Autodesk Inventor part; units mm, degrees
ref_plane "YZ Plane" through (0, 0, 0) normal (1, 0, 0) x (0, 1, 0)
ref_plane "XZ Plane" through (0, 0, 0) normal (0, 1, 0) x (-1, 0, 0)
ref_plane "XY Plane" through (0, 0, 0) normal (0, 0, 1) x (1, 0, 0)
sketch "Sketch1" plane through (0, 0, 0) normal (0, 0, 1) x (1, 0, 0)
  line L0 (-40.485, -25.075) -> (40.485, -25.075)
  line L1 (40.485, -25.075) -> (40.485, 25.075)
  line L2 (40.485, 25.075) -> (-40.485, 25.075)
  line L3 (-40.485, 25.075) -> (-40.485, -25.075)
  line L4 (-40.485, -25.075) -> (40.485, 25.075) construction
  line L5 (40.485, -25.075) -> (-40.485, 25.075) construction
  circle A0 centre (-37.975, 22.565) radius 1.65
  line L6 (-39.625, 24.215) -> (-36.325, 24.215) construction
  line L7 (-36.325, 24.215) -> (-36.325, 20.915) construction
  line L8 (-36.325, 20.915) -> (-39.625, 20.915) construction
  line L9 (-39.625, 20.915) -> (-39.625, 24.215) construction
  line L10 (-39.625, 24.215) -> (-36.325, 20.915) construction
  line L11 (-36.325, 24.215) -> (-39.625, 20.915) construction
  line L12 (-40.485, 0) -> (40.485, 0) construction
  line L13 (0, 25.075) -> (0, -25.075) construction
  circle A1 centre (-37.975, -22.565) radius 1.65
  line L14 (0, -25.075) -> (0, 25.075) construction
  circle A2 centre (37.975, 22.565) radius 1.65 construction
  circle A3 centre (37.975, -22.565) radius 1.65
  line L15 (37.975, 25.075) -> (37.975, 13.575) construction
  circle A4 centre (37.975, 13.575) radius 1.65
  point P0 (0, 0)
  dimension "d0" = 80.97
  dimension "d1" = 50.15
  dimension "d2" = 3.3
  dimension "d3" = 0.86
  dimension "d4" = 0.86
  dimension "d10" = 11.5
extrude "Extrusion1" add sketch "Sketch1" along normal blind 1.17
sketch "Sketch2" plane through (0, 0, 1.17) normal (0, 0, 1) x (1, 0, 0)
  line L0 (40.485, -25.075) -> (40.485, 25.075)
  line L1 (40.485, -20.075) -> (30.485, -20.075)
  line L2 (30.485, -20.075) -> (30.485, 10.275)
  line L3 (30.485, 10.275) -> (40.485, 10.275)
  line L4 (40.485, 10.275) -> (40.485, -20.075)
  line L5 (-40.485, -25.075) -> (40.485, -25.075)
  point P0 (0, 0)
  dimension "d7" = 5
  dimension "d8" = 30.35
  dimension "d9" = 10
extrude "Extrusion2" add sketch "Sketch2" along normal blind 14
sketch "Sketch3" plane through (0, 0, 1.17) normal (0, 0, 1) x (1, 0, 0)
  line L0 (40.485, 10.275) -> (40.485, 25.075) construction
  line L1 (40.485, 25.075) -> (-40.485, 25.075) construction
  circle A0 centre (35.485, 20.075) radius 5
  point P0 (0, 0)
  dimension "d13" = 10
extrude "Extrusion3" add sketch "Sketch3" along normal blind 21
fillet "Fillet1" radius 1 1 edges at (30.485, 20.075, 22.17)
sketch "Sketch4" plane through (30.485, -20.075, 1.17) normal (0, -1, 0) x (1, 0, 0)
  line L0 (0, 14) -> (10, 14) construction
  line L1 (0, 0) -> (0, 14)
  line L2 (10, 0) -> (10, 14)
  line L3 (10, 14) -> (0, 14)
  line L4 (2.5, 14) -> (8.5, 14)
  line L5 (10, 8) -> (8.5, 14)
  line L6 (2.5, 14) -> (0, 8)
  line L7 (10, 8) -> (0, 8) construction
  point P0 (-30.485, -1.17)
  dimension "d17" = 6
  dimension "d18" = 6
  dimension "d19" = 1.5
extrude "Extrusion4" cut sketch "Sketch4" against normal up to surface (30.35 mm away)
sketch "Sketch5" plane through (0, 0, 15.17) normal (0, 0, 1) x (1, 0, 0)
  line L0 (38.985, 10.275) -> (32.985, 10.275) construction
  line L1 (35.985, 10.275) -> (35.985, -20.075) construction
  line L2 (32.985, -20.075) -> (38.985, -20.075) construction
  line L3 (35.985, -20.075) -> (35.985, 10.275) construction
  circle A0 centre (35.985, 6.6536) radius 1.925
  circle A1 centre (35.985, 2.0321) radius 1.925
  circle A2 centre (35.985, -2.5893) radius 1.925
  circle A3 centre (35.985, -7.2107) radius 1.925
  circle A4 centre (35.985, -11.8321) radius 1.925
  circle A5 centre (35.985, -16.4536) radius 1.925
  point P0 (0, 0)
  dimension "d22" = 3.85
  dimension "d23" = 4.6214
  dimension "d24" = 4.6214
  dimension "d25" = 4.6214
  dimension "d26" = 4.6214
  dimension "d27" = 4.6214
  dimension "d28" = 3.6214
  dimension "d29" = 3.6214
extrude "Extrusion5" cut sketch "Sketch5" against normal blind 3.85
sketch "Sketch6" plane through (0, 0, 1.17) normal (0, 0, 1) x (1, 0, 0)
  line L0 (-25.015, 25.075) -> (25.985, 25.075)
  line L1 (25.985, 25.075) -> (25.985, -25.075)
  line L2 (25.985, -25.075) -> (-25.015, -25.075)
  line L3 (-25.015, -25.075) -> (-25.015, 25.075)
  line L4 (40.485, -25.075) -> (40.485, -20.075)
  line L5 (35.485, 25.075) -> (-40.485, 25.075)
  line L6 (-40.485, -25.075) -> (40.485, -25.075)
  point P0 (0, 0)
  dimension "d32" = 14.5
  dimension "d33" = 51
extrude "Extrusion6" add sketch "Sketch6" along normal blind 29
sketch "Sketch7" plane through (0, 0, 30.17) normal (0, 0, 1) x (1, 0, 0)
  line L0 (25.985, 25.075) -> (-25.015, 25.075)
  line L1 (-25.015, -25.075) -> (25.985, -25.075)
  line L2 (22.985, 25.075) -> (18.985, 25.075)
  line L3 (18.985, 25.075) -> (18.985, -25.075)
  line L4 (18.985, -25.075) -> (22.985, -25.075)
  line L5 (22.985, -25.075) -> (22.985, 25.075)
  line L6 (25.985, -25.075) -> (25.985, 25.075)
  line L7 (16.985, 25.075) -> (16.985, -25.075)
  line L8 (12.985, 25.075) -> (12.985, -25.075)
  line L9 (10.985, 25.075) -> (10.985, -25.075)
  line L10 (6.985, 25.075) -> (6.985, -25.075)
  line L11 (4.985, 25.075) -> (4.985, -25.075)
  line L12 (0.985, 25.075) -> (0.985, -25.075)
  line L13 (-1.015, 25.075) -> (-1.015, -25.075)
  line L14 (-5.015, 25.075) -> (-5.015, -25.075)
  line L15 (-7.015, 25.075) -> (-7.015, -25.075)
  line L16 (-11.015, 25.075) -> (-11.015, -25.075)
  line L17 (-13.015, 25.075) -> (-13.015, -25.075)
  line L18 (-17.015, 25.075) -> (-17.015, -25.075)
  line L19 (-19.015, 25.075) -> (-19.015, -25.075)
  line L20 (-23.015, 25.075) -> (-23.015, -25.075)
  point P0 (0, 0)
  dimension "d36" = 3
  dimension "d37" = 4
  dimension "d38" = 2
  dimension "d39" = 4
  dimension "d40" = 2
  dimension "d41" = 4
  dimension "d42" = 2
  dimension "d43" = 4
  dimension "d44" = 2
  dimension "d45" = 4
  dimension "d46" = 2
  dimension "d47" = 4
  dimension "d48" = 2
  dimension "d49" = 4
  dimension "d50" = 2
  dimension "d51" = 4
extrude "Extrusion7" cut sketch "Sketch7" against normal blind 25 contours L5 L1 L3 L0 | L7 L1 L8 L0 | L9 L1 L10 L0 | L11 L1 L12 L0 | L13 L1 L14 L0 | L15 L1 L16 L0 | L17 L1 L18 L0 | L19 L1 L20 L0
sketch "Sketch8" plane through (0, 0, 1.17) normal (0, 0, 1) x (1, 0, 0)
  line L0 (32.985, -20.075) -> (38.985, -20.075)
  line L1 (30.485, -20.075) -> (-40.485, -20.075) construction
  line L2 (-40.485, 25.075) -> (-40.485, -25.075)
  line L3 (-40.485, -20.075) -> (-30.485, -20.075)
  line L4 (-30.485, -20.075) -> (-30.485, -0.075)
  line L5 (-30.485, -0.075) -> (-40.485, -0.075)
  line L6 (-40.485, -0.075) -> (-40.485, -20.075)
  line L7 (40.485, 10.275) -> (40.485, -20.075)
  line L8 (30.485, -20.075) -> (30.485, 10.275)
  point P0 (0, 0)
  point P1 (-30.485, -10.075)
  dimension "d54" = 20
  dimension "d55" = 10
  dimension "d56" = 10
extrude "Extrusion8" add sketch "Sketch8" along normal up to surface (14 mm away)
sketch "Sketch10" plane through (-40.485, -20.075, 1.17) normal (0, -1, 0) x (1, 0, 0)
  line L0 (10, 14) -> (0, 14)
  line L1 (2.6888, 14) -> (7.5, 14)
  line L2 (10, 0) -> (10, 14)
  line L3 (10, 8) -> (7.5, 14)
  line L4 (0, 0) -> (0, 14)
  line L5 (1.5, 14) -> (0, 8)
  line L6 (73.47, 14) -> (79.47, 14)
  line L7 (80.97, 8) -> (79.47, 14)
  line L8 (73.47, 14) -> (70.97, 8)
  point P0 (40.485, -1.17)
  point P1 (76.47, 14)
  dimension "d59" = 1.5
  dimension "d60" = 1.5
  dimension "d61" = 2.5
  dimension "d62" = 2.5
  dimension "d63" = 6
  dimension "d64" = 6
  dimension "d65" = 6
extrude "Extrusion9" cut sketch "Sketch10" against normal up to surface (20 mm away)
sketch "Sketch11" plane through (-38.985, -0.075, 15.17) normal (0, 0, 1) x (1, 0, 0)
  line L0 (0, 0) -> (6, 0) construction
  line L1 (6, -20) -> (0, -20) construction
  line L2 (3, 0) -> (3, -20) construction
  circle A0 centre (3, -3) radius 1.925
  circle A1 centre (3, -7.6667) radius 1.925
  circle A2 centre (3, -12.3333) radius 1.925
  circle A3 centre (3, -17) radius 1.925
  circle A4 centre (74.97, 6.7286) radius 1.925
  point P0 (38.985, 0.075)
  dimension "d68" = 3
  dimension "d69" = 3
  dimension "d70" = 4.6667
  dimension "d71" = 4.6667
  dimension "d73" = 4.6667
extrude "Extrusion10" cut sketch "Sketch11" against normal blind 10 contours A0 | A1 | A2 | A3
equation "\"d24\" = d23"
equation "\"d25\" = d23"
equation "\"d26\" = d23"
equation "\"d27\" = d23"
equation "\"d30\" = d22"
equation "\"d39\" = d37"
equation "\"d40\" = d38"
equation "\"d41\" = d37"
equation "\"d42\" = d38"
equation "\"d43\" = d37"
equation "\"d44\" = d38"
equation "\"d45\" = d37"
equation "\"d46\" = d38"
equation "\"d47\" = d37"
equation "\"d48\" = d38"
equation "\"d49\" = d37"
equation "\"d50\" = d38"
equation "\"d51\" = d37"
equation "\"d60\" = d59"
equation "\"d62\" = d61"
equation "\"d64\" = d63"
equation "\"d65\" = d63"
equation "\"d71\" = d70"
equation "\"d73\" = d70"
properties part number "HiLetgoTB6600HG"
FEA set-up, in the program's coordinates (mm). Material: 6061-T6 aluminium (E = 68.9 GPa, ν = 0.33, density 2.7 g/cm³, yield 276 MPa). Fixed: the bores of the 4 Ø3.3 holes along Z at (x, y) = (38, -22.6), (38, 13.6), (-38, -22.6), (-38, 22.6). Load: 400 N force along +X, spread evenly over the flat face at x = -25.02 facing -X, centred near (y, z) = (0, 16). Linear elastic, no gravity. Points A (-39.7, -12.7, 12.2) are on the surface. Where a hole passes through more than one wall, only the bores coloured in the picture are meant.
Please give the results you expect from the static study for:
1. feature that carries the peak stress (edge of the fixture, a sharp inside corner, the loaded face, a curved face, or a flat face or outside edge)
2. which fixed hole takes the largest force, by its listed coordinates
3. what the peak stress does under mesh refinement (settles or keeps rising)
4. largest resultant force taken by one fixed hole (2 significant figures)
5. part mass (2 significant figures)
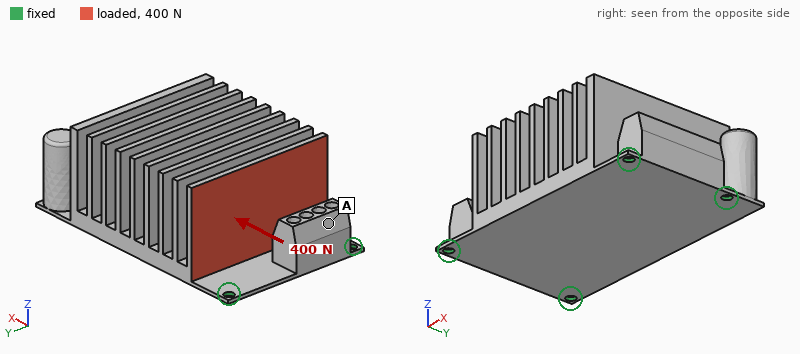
edge of the fixture
(38, 13.6)
keeps rising
240 N
120 g
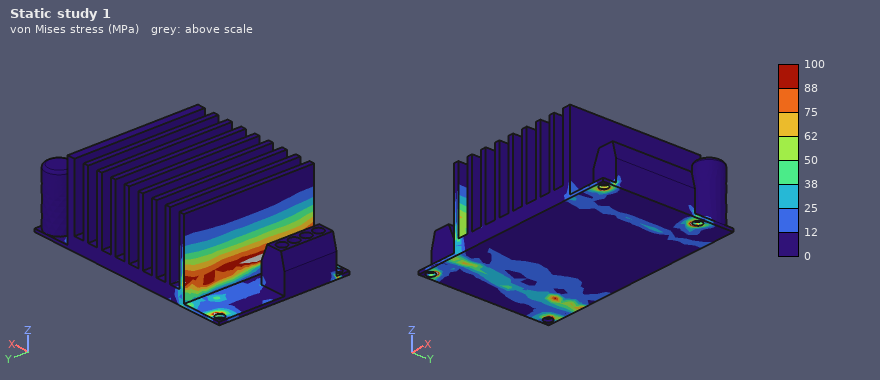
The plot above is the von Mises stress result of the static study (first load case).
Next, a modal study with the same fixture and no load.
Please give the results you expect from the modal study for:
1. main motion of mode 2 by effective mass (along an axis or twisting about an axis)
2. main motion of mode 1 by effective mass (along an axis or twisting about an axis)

along Y
along Z
